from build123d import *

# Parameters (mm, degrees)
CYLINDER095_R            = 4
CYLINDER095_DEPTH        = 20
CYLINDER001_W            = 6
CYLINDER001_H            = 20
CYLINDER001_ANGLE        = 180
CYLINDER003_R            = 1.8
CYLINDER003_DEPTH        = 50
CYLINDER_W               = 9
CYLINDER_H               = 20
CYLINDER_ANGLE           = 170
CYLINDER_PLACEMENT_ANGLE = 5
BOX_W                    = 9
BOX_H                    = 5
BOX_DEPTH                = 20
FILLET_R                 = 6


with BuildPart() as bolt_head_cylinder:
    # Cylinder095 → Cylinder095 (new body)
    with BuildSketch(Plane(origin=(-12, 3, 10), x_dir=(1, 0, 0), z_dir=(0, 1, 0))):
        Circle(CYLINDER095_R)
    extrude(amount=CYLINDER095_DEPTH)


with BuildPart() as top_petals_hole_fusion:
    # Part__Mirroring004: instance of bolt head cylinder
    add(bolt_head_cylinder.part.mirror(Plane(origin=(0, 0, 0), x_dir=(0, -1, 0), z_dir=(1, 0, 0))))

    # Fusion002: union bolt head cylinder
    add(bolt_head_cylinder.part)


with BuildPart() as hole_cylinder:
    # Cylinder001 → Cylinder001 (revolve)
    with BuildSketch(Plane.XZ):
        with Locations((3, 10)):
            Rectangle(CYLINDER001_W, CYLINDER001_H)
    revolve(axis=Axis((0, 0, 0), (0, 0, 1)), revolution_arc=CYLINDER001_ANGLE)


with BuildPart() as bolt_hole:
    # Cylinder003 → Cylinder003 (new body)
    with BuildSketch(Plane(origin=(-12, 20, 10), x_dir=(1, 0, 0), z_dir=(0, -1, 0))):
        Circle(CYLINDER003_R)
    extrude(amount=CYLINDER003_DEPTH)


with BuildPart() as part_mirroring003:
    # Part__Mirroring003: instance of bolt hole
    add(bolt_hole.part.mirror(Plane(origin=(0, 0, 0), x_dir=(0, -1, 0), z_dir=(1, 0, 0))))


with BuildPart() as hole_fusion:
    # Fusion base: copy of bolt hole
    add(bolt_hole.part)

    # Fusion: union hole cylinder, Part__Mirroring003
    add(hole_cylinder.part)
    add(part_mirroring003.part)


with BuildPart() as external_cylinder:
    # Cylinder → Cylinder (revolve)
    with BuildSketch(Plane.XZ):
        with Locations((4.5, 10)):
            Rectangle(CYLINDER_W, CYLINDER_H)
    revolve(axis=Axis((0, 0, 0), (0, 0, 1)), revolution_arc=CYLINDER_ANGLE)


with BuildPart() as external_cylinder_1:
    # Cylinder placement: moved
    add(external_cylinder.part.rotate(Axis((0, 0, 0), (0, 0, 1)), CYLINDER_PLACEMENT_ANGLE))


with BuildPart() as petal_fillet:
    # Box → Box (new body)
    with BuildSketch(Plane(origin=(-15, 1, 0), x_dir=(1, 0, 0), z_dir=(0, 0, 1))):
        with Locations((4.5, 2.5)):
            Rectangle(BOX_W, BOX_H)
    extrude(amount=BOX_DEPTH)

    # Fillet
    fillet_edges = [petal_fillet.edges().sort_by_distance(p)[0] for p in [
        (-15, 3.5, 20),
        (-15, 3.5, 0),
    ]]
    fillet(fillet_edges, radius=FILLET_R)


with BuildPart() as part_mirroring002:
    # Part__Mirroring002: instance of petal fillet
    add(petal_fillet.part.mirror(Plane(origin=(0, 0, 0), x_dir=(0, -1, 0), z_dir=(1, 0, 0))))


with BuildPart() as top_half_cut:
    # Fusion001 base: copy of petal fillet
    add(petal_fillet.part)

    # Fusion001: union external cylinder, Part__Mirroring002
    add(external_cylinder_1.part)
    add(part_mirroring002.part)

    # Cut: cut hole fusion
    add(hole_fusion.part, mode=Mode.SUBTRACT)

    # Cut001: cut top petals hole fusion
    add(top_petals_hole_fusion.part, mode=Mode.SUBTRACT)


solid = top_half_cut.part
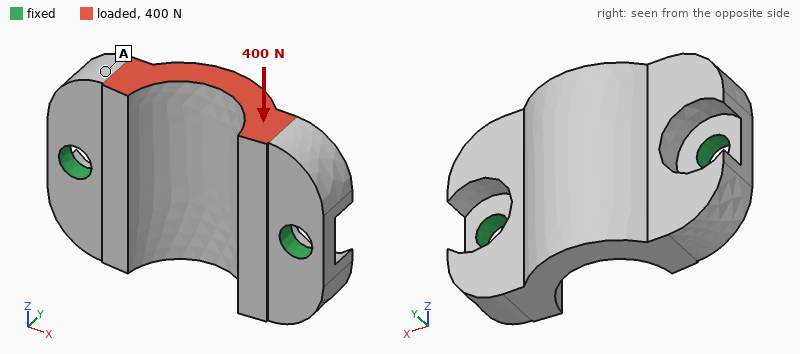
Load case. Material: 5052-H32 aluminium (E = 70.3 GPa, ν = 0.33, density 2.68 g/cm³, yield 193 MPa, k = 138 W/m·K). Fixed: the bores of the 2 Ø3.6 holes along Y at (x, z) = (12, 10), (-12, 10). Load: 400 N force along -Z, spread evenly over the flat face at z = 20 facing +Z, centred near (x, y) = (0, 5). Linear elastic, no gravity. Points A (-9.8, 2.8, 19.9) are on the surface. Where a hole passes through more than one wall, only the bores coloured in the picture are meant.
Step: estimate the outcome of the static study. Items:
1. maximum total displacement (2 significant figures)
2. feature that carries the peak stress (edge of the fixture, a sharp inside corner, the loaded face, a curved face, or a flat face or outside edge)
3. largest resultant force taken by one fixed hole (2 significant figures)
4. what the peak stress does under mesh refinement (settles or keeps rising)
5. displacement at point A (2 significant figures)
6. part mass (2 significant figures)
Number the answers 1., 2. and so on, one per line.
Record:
1. 20 µm
2. edge of the fixture
3. 200 N
4. keeps rising
5. 12 µm
6. 6.0 g
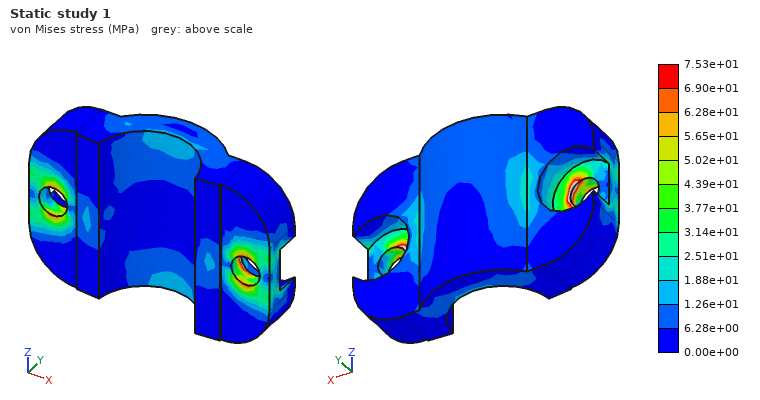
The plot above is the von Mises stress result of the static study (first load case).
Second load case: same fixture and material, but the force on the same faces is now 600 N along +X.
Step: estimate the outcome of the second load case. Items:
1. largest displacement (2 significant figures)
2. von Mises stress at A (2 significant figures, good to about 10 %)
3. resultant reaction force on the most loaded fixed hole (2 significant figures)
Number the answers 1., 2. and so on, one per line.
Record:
1. 11 µm
2. 13 MPa
3. 370 N
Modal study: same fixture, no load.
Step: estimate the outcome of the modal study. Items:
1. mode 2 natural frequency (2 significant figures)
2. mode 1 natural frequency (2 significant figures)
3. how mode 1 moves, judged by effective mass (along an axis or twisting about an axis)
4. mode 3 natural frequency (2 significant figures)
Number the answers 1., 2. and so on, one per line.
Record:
1. 25 kHz
2. 10 kHz
3. along Z
4. 25 kHz
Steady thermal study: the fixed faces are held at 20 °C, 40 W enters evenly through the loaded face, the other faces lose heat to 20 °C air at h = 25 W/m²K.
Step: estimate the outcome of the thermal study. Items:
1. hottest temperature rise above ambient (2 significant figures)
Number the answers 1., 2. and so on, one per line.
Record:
1. 49 K
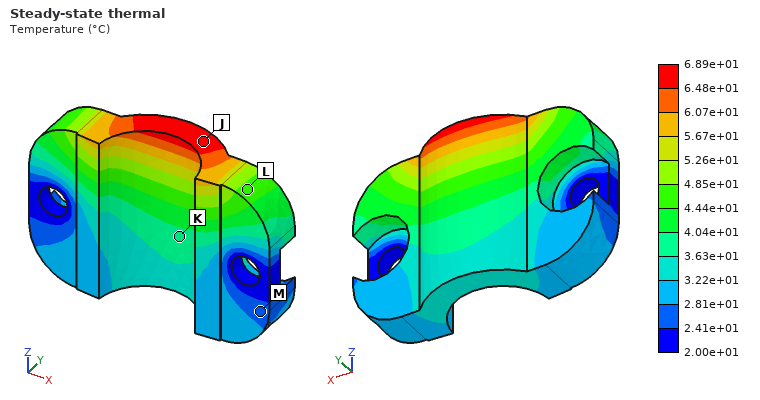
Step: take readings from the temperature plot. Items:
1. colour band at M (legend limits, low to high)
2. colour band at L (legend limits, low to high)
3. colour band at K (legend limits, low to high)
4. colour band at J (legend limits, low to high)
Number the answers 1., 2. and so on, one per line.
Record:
1. 2.41e+01 to 2.81e+01 °C
2. 4.44e+01 to 4.85e+01 °C
3. 3.63e+01 to 4.04e+01 °C
4. 6.48e+01 to 6.89e+01 °C
